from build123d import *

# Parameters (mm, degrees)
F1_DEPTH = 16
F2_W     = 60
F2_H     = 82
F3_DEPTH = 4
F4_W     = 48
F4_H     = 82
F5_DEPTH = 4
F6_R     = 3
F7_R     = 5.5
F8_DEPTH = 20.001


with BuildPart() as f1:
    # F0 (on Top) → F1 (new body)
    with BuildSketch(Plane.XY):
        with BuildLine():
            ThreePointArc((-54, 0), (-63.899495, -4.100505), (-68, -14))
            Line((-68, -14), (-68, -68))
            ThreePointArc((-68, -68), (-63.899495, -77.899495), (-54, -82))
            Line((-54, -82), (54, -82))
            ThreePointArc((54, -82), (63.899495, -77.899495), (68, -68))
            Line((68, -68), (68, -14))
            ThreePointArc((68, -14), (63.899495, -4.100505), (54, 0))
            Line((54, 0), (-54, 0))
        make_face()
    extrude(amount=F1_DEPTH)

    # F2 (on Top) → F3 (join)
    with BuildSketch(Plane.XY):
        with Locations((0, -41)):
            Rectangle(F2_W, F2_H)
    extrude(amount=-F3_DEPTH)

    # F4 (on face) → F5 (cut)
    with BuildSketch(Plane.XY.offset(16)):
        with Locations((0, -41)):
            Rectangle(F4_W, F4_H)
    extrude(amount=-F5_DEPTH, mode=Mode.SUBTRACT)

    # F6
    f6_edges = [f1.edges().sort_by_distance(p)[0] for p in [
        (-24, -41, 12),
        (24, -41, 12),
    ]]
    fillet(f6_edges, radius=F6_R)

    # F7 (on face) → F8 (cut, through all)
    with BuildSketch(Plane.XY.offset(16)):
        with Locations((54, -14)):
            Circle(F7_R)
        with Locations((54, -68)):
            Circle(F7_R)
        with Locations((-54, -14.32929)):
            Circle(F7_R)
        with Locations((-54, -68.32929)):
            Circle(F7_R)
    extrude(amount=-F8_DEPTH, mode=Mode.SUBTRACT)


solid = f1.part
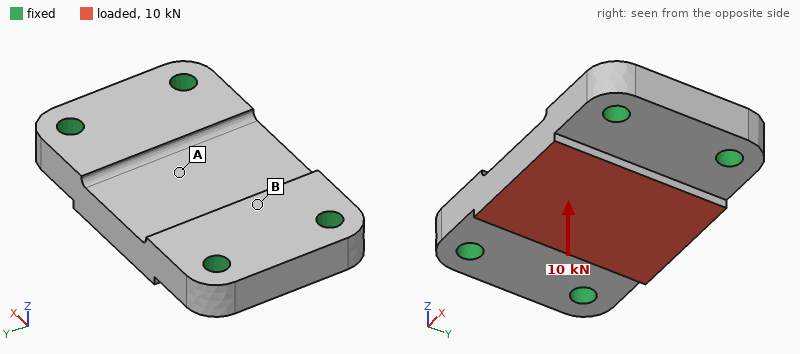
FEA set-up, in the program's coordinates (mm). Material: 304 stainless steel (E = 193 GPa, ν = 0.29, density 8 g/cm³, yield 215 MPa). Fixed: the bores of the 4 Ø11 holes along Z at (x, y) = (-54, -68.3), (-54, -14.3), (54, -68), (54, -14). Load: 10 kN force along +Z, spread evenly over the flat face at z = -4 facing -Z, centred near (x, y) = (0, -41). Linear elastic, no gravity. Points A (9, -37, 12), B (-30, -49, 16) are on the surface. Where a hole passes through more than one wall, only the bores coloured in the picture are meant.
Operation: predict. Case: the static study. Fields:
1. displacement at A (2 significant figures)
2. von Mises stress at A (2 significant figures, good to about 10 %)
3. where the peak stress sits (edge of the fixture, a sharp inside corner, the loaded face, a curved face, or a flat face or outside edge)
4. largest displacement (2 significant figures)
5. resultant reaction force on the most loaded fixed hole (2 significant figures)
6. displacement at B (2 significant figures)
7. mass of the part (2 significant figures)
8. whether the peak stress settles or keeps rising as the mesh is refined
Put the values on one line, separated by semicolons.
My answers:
9.8 µm; 13 MPa; edge of the fixture; 11 µm; 3.3 kN; 6.0 µm; 1.4 kg; keeps rising
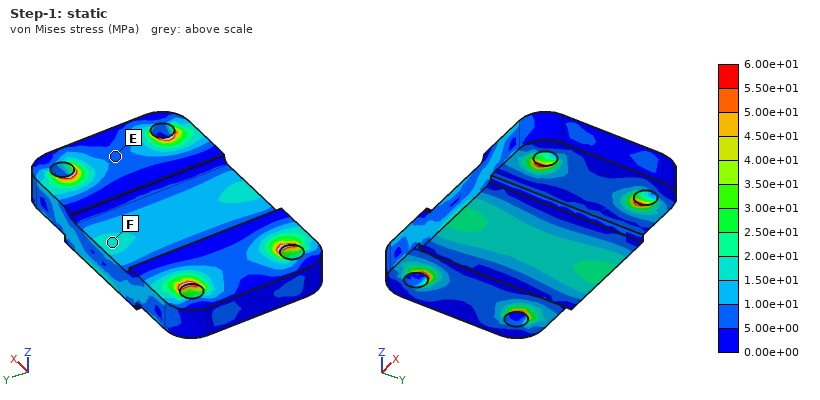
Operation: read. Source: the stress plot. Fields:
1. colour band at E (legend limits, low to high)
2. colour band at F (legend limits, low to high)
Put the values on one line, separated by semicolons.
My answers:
5.00e+00 to 1.00e+01 MPa; 1.50e+01 to 2.00e+01 MPa
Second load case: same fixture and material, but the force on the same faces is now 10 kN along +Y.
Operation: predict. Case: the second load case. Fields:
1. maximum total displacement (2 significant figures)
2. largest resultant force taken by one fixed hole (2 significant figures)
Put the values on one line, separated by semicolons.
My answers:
6.8 µm; 3.5 kN
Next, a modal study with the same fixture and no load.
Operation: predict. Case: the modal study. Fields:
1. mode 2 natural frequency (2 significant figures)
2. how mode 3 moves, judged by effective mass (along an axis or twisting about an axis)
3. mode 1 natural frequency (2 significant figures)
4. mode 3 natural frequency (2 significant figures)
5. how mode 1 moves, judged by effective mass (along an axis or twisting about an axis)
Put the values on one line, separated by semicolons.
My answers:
8200 Hz; along Y; 6300 Hz; 12 kHz; along Z
